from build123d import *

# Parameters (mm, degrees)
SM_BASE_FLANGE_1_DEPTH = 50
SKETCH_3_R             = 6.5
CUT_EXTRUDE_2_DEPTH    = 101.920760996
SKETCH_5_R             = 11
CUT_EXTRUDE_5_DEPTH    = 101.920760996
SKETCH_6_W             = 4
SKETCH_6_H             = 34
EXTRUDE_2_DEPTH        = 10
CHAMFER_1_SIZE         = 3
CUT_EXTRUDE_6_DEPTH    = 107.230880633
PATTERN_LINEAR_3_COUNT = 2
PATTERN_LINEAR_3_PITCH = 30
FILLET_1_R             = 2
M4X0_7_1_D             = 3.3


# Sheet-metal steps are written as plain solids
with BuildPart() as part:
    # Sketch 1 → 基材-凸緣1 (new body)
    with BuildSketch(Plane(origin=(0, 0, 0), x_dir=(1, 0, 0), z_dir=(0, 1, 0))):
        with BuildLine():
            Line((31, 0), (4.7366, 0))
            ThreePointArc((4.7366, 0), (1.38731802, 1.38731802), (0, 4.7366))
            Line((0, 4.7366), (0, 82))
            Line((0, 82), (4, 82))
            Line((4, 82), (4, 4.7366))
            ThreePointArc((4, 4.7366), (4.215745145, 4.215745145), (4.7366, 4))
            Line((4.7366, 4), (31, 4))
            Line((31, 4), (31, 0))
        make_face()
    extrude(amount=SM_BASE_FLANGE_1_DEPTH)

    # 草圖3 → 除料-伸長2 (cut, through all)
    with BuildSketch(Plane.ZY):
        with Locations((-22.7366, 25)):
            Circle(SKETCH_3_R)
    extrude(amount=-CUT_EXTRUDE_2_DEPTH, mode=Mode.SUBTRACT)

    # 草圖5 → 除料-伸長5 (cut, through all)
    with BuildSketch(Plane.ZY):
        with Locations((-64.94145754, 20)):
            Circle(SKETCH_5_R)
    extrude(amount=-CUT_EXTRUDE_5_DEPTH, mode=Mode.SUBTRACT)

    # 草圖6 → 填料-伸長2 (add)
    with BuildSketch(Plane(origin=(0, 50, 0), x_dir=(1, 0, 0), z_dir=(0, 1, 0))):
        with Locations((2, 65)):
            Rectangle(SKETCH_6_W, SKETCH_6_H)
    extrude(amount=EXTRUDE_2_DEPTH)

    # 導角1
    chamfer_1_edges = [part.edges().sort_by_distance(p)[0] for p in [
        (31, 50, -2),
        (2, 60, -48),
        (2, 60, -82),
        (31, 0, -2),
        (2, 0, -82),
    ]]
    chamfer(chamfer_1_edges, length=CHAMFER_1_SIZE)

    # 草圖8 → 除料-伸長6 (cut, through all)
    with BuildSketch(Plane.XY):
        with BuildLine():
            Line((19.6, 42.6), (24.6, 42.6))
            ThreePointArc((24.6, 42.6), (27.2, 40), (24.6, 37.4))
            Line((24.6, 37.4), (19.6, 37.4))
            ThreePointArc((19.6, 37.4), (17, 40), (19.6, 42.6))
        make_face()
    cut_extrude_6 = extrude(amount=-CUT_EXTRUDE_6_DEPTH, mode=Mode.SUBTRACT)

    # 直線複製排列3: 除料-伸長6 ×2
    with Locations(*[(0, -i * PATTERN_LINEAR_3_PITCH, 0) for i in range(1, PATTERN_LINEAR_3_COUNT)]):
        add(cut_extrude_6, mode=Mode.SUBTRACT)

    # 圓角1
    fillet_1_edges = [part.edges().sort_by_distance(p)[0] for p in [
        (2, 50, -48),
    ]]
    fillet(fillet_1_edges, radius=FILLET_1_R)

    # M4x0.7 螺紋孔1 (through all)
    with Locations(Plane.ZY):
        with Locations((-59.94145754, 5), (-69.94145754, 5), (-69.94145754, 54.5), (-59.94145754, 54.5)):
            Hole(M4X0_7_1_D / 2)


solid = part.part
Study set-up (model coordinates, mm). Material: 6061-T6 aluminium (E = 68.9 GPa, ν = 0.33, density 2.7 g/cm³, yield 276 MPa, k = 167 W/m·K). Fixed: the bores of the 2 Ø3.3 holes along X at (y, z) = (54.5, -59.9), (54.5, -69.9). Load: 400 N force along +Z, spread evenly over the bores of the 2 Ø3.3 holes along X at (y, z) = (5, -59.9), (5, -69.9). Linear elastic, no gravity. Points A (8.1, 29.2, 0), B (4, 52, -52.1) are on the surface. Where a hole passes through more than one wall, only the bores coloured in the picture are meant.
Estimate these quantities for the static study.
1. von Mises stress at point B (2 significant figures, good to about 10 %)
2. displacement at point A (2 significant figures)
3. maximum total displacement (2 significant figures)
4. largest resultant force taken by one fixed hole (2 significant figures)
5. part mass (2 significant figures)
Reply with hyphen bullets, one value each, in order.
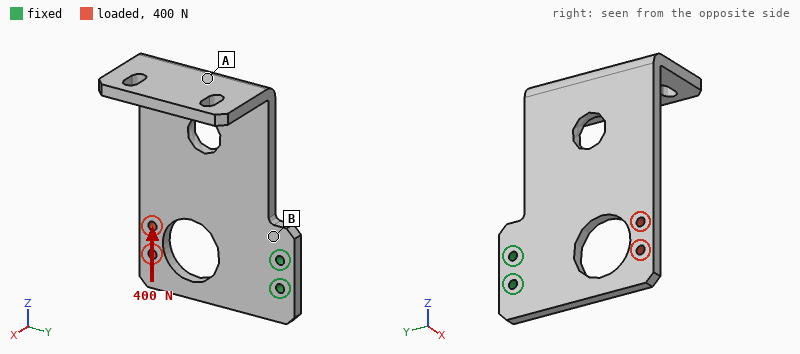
- 17 MPa
- 0.087 mm
- 0.11 mm
- 1.5 kN
- 55 g
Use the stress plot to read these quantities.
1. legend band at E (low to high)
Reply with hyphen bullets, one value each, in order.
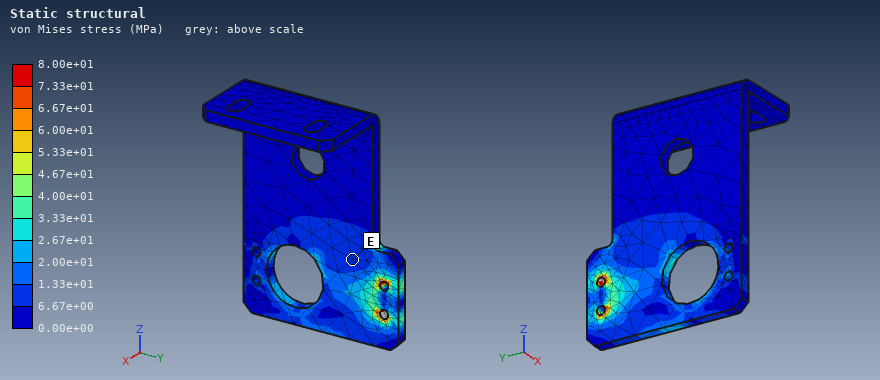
- 6.67e+00 to 1.33e+01 MPa
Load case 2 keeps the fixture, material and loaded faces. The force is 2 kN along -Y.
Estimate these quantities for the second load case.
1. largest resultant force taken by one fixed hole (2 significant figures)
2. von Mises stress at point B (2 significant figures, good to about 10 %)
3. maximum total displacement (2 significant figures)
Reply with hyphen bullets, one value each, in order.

- 1.0 kN
- 12 MPa
- 42 µm
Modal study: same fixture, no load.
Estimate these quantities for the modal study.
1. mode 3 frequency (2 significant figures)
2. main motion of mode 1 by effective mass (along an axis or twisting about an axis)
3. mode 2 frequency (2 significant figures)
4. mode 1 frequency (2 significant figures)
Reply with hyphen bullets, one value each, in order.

- 1600 Hz
- along X
- 770 Hz
- 340 Hz
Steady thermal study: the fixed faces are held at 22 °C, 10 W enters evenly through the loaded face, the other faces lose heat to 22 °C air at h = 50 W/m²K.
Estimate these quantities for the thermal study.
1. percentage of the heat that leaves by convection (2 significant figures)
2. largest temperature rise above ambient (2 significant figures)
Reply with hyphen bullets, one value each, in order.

- 42 %
- 24 K
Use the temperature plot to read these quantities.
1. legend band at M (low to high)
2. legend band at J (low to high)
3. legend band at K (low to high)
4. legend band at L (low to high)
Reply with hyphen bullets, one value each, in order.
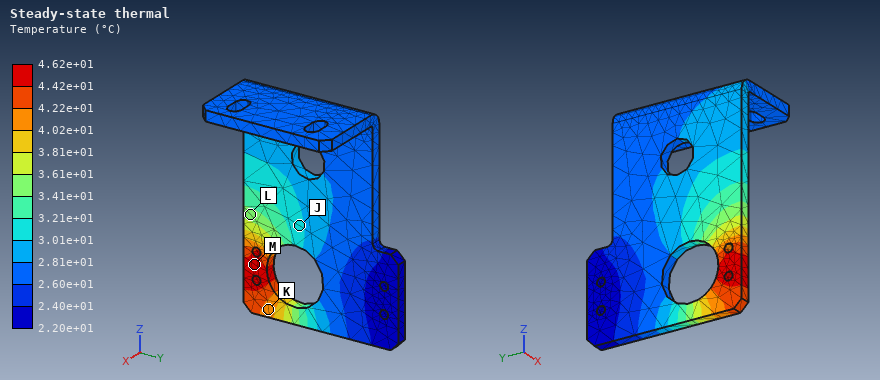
- 4.42e+01 to 4.62e+01 °C
- 3.01e+01 to 3.21e+01 °C
- 4.02e+01 to 4.22e+01 °C
- 3.41e+01 to 3.61e+01 °C
